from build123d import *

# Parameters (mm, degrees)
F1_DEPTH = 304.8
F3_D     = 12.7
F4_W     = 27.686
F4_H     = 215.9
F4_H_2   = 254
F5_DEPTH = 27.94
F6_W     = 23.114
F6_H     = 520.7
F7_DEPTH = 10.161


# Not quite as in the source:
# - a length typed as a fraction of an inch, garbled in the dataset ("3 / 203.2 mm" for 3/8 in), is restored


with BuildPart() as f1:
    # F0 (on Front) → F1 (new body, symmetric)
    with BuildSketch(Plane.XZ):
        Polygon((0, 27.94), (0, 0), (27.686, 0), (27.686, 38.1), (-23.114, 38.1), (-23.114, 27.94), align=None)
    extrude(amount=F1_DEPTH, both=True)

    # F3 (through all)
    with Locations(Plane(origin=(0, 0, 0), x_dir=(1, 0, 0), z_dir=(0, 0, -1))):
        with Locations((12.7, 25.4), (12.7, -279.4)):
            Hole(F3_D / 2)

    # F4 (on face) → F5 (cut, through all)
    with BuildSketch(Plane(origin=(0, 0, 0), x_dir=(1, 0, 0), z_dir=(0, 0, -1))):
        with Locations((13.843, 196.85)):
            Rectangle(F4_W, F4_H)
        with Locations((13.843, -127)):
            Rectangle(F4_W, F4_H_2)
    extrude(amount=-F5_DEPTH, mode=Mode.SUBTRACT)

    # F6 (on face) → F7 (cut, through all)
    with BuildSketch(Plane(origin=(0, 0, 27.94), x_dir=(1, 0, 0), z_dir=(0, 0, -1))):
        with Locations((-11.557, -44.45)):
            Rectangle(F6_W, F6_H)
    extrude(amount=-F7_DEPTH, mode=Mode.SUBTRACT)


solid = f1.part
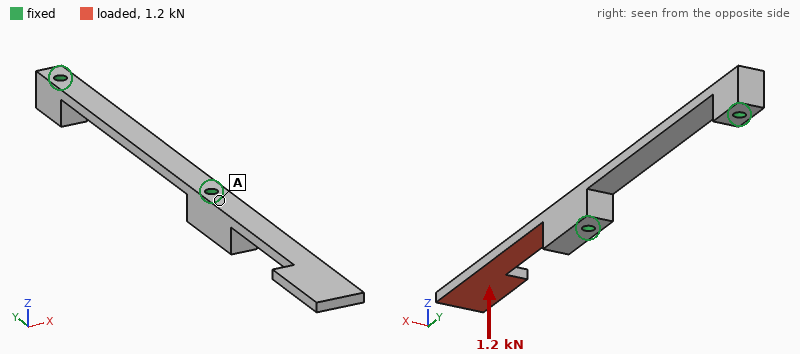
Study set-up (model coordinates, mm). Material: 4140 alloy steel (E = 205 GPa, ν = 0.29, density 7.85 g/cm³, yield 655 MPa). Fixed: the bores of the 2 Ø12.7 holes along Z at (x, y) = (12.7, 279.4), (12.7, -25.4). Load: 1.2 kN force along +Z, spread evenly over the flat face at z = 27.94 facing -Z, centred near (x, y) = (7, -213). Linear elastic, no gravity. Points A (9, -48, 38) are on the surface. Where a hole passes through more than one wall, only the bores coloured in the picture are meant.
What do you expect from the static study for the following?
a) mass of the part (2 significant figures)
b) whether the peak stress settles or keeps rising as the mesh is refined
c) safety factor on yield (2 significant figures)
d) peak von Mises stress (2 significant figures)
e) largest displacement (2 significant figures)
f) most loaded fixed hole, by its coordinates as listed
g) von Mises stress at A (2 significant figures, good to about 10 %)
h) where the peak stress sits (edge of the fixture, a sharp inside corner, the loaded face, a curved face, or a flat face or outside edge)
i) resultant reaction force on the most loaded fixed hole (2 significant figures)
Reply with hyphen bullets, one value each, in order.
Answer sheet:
- 2.3 kg
- settles
- 2.2
- 300 MPa
- 4.2 mm
- (12.7, -25.4)
- 31 MPa
- a flat face or outside edge
- 1.2 kN
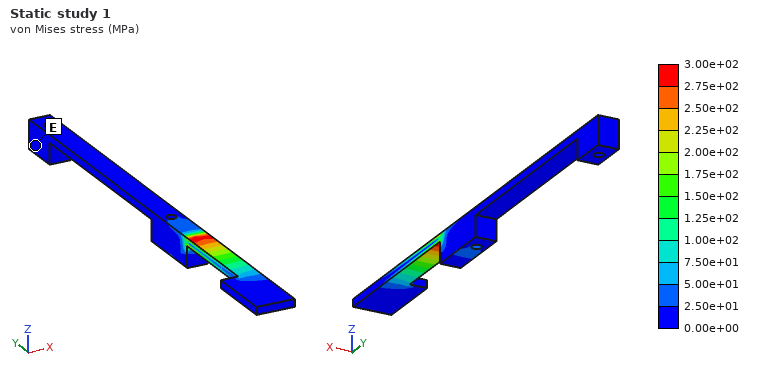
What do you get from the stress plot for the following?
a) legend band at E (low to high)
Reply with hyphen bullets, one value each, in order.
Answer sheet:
- 0.00e+00 to 2.50e+01 MPa
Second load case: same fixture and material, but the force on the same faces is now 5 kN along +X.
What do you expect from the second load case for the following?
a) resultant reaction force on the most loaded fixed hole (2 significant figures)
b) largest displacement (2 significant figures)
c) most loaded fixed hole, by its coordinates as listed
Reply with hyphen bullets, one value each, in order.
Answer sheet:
- 5.1 kN
- 3.5 mm
- (12.7, -25.4)
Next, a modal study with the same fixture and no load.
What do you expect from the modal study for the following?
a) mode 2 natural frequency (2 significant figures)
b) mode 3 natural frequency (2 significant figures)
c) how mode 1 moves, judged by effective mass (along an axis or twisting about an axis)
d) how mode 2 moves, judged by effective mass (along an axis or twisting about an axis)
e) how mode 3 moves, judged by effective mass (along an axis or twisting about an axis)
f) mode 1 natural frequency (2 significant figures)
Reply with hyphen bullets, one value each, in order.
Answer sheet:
- 290 Hz
- 750 Hz
- along Z
- along X
- along Z
- 130 Hz
